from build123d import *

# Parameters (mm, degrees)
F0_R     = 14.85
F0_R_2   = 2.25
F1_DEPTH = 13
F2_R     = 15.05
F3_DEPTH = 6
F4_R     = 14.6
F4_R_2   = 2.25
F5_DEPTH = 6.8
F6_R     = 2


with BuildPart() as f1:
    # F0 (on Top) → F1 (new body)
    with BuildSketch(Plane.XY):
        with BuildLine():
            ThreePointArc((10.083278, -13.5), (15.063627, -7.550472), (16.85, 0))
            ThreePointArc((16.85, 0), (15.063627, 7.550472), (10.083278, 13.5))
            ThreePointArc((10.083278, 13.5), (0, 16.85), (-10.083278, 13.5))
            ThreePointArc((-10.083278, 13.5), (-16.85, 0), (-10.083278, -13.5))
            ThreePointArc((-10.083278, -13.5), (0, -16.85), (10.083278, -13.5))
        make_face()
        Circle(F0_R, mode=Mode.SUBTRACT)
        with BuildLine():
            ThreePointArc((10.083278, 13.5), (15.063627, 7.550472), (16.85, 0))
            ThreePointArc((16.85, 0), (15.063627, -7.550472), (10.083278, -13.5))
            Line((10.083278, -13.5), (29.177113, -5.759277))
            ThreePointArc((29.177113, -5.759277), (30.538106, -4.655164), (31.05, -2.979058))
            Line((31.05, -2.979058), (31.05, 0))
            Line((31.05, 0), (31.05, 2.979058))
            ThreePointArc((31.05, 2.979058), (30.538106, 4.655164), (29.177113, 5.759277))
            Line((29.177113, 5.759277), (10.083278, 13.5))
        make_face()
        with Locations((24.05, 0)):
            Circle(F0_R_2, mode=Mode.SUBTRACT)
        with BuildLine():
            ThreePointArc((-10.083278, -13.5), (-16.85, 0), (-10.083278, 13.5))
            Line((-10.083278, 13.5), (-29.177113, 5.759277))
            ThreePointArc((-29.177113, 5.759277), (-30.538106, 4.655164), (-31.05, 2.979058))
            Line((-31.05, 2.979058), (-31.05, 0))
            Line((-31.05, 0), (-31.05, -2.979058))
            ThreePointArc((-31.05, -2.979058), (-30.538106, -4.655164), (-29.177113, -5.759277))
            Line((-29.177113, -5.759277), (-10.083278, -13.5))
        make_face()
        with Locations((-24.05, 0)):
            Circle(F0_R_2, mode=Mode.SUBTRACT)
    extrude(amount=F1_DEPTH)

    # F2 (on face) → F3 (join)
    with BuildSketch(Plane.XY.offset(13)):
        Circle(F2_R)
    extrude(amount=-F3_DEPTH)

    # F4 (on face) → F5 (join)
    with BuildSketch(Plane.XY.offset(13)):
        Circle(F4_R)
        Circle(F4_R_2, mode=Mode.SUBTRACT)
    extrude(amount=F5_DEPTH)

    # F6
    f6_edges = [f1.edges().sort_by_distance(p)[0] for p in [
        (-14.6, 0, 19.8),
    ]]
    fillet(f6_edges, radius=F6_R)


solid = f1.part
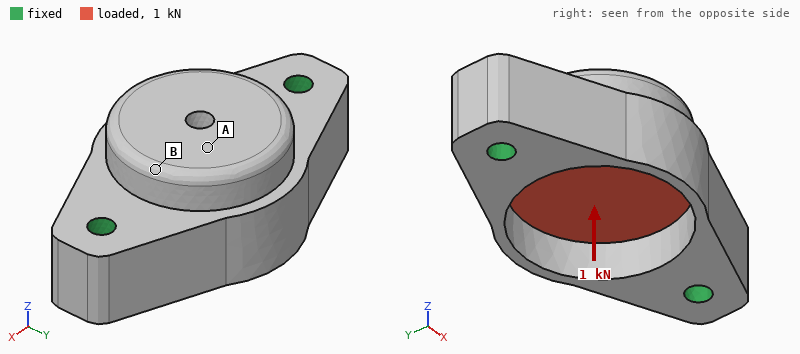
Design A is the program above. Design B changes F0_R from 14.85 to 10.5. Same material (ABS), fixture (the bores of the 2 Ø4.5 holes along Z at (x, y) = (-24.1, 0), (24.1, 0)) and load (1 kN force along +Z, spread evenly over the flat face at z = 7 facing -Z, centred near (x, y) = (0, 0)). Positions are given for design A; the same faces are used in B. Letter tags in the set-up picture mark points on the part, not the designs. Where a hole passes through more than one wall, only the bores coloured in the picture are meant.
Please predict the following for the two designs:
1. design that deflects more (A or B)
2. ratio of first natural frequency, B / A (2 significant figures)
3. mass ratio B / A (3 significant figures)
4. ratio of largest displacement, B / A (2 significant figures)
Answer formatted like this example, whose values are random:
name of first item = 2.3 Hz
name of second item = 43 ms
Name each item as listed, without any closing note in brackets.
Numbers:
design that deflects more = A
ratio of first natural frequency, B / A = 1.0
mass ratio B / A = 1.14
ratio of largest displacement, B / A = 0.78
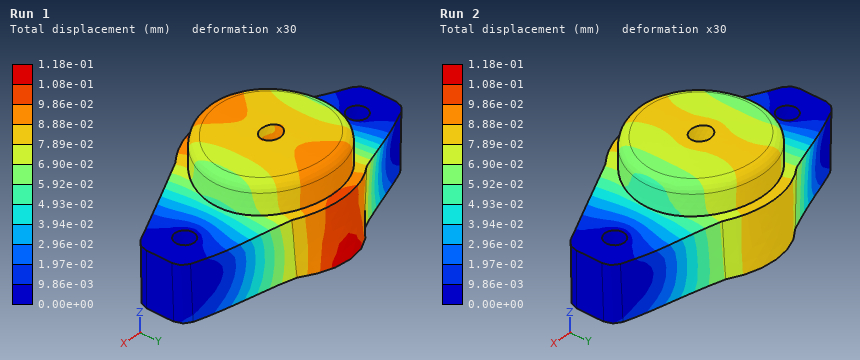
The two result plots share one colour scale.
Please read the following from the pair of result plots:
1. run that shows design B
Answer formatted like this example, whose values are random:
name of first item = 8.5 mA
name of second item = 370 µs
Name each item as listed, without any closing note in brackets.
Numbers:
run that shows design B = Run 2
